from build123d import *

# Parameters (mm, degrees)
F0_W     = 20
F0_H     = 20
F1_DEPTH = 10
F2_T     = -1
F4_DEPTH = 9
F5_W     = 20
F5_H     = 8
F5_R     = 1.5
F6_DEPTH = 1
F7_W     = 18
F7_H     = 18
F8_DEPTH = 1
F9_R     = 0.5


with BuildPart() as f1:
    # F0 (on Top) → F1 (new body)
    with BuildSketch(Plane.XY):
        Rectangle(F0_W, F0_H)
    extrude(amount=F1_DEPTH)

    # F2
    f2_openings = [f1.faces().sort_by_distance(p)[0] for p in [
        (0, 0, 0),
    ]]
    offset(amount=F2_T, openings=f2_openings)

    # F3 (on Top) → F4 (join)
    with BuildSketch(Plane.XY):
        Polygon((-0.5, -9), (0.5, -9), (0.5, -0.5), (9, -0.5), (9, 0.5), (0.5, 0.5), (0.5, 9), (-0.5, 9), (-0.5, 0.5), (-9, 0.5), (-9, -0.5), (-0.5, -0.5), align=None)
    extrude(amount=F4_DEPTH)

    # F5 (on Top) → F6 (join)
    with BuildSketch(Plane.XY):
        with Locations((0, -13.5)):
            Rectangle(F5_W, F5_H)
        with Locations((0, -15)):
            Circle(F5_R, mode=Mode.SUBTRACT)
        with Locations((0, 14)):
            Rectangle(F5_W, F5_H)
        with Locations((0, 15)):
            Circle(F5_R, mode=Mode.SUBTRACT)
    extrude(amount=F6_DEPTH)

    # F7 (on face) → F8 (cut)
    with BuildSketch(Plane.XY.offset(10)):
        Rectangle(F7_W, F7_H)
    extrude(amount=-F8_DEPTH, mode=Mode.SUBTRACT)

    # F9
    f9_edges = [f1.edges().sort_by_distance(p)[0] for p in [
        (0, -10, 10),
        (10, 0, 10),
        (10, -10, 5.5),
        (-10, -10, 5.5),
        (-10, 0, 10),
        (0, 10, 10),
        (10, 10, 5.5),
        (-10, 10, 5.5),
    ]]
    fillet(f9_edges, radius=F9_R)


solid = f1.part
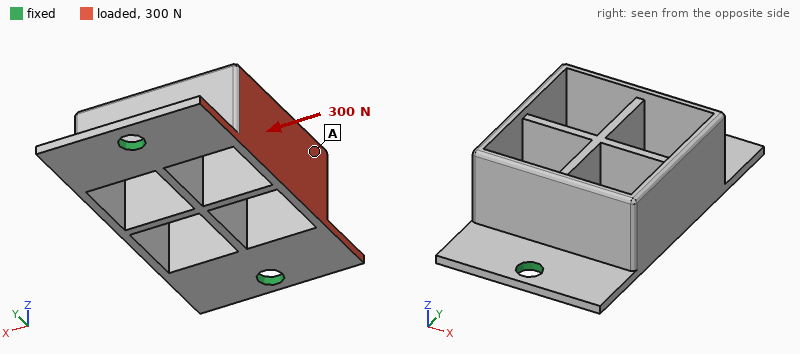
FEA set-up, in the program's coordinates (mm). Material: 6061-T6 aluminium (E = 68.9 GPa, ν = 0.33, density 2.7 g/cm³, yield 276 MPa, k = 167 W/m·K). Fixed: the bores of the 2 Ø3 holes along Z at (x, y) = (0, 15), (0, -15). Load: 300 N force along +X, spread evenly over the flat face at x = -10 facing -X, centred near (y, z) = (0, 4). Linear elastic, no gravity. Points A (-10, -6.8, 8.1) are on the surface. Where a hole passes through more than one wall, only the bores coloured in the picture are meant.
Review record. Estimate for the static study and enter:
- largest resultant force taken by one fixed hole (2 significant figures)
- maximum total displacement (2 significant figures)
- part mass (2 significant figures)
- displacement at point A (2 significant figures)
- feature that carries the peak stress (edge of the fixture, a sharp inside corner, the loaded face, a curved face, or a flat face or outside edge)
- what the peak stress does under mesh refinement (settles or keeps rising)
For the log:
150 N
0.21 mm
3.7 g
0.18 mm
edge of the fixture
keeps rising
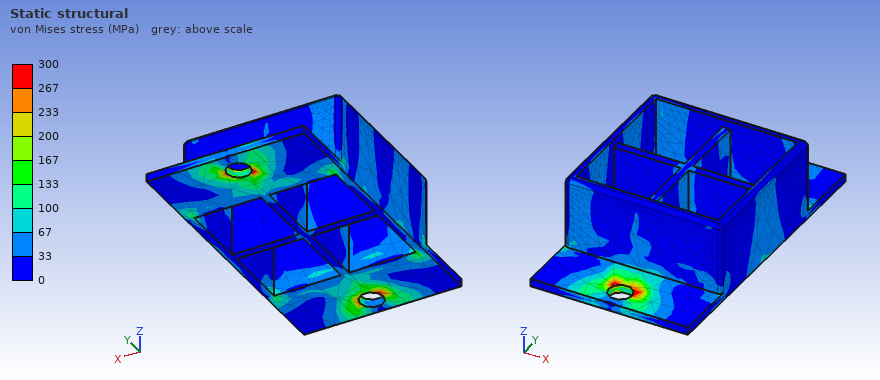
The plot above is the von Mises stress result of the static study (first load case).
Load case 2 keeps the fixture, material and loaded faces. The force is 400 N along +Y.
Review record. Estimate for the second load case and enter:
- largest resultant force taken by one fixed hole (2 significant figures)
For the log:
220 N
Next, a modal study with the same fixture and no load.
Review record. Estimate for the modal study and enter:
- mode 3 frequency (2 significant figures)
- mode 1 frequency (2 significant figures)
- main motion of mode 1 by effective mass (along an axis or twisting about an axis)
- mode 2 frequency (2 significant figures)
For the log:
9000 Hz
3200 Hz
along X
9000 Hz
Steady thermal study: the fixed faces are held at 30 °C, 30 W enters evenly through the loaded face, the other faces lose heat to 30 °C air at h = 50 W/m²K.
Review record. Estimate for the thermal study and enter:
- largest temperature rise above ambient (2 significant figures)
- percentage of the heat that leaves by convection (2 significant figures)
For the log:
85 K
16 %
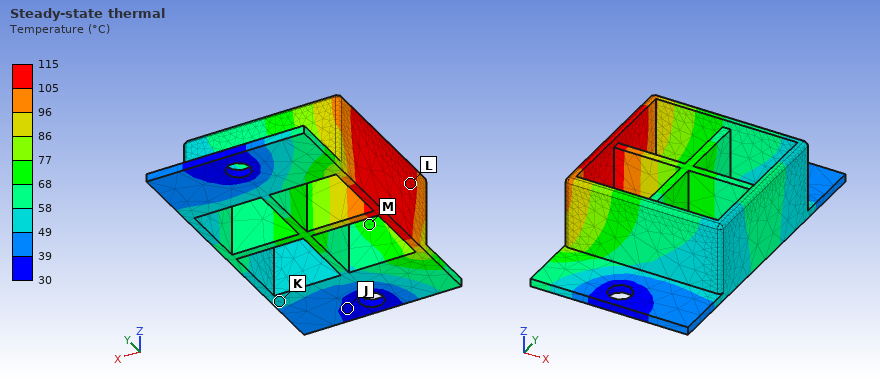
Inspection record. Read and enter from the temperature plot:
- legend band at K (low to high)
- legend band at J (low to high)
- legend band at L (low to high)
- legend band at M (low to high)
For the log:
49 to 58 °C
30 to 39 °C
105 to 115 °C
68 to 77 °C
